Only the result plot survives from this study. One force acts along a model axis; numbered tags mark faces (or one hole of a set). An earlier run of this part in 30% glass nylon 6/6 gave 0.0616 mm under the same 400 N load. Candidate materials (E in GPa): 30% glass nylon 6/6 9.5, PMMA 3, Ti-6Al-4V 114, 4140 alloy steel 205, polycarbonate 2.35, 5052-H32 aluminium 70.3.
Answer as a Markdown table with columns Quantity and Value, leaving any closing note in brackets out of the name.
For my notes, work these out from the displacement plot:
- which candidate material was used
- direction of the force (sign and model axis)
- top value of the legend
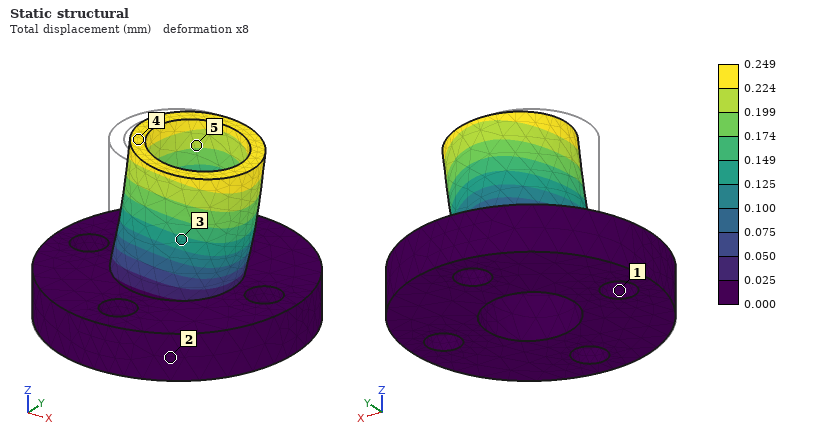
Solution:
| Quantity | Value |
|---|---|
| which candidate material was used | polycarbonate |
| direction of the force | +X |
| top value of the legend | 0.249 mm |
